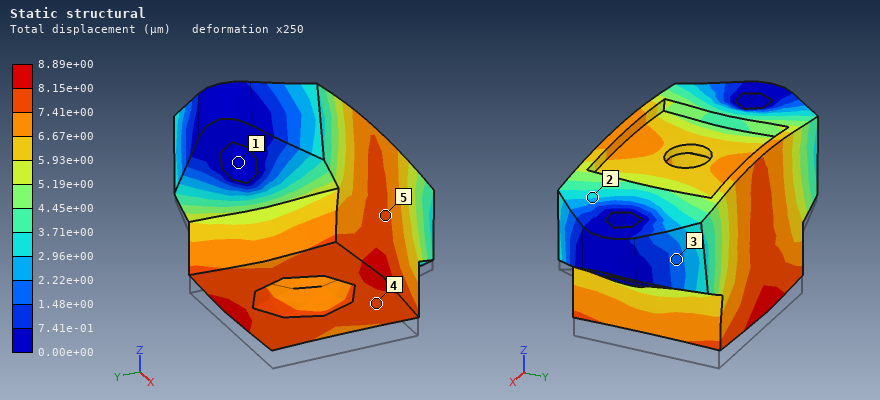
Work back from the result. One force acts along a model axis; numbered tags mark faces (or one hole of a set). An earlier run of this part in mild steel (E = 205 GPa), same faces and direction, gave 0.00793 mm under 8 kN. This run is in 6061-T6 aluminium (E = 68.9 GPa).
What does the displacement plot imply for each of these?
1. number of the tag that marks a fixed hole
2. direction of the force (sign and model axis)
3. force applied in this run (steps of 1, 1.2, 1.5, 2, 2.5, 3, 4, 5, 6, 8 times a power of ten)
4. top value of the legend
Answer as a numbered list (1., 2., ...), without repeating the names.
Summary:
1. 1
2. +Z
3. 3 kN
4. 8.89e+00 µm
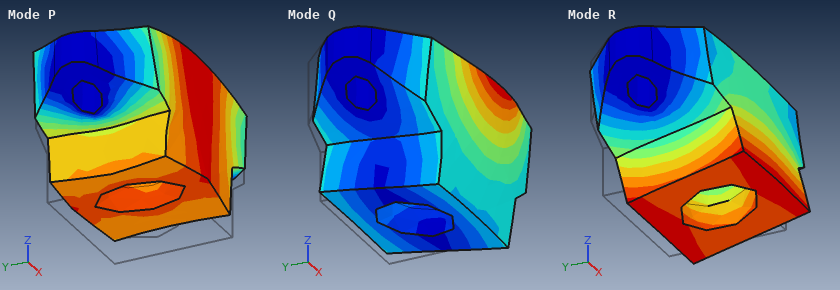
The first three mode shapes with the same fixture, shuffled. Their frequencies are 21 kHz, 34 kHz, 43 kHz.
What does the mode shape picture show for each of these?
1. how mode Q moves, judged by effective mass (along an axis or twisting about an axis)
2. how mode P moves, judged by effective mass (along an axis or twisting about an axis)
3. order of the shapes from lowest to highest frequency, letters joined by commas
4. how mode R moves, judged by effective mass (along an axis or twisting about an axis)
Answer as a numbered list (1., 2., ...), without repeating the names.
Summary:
1. along Y
2. along Z
3. R, P, Q
4. along Y
